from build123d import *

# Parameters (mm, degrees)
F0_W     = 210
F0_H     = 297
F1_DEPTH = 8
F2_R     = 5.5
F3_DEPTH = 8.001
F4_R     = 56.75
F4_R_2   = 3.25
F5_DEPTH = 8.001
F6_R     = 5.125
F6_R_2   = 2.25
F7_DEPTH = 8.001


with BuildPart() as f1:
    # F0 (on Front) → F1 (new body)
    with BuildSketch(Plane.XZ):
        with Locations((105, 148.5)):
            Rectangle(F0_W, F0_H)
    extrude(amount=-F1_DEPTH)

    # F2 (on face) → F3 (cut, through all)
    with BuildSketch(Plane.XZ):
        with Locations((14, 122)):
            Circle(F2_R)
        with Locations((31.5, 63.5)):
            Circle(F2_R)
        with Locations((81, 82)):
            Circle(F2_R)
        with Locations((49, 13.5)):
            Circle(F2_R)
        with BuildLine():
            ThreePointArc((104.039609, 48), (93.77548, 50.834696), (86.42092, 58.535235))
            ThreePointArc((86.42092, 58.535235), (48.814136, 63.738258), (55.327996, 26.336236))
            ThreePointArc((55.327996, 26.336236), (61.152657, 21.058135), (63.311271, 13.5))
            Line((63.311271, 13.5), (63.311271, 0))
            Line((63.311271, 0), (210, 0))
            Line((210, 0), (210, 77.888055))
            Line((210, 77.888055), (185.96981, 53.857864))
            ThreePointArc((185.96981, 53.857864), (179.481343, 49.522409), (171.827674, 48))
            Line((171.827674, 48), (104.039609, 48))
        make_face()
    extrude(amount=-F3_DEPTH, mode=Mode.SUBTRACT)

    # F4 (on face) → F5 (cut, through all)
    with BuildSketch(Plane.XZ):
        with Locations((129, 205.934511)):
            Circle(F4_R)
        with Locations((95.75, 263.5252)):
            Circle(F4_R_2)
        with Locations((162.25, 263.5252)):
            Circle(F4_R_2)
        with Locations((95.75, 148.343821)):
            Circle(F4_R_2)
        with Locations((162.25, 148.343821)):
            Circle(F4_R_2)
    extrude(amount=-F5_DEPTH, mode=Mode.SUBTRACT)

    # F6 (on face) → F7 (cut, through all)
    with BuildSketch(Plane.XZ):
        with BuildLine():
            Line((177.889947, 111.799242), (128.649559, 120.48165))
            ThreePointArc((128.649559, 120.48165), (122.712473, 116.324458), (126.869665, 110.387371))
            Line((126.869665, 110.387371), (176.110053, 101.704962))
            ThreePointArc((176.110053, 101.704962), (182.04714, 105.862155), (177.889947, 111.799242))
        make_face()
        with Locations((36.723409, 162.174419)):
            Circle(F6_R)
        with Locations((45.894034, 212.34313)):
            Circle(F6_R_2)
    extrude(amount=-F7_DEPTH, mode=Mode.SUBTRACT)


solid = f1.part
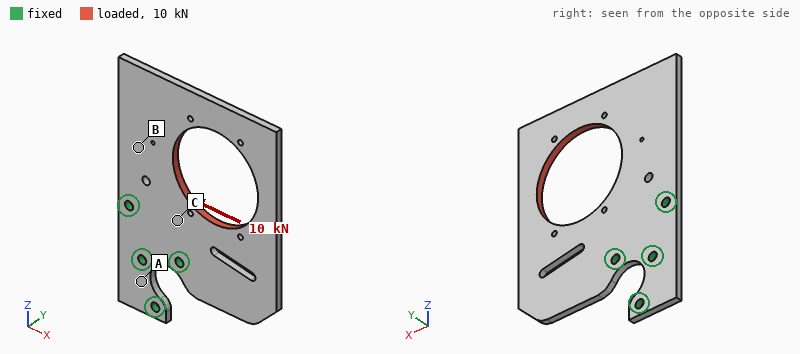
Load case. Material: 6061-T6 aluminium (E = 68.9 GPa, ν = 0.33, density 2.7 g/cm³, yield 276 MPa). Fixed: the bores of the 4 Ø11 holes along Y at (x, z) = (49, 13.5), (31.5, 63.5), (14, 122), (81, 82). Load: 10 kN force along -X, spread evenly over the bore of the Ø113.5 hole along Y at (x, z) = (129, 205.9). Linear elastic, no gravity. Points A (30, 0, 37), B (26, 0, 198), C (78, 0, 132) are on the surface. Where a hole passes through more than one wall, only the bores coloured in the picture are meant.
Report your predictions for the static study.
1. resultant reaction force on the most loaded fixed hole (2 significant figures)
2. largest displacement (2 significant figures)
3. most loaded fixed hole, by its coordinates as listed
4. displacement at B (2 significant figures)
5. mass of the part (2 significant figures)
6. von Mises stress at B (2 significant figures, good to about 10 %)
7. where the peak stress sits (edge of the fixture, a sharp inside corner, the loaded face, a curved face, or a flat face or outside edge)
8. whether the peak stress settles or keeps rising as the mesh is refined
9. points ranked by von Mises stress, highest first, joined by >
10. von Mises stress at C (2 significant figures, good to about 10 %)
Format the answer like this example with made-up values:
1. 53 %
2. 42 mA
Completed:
1. 15 kN
2. 0.32 mm
3. (14, 122)
4. 0.11 mm
5. 910 g
6. 17 MPa
7. edge of the fixture
8. keeps rising
9. C > B > A
10. 42 MPa
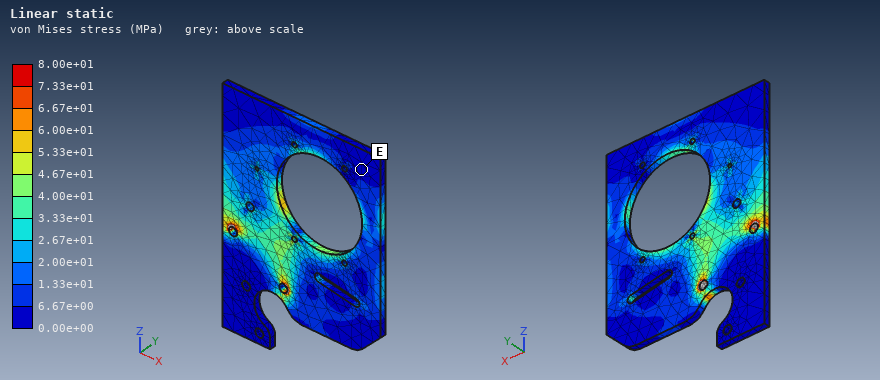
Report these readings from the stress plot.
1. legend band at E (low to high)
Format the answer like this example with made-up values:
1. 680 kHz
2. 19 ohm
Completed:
1. 0.00e+00 to 6.67e+00 MPa
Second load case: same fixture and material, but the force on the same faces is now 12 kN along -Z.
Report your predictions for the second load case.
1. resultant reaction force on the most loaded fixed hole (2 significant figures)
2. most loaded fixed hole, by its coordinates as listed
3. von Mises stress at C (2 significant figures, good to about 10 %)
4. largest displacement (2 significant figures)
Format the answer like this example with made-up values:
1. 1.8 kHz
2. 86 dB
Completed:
1. 16 kN
2. (81, 82)
3. 39 MPa
4. 0.31 mm
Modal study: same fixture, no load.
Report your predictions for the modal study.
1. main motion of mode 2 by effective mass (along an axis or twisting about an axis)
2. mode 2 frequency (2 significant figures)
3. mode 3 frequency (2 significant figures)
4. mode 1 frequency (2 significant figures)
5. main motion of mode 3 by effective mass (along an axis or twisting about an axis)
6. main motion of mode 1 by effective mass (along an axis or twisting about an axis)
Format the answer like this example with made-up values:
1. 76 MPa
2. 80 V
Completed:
1. twisting about Z
2. 280 Hz
3. 480 Hz
4. 140 Hz
5. along Y
6. along Y
